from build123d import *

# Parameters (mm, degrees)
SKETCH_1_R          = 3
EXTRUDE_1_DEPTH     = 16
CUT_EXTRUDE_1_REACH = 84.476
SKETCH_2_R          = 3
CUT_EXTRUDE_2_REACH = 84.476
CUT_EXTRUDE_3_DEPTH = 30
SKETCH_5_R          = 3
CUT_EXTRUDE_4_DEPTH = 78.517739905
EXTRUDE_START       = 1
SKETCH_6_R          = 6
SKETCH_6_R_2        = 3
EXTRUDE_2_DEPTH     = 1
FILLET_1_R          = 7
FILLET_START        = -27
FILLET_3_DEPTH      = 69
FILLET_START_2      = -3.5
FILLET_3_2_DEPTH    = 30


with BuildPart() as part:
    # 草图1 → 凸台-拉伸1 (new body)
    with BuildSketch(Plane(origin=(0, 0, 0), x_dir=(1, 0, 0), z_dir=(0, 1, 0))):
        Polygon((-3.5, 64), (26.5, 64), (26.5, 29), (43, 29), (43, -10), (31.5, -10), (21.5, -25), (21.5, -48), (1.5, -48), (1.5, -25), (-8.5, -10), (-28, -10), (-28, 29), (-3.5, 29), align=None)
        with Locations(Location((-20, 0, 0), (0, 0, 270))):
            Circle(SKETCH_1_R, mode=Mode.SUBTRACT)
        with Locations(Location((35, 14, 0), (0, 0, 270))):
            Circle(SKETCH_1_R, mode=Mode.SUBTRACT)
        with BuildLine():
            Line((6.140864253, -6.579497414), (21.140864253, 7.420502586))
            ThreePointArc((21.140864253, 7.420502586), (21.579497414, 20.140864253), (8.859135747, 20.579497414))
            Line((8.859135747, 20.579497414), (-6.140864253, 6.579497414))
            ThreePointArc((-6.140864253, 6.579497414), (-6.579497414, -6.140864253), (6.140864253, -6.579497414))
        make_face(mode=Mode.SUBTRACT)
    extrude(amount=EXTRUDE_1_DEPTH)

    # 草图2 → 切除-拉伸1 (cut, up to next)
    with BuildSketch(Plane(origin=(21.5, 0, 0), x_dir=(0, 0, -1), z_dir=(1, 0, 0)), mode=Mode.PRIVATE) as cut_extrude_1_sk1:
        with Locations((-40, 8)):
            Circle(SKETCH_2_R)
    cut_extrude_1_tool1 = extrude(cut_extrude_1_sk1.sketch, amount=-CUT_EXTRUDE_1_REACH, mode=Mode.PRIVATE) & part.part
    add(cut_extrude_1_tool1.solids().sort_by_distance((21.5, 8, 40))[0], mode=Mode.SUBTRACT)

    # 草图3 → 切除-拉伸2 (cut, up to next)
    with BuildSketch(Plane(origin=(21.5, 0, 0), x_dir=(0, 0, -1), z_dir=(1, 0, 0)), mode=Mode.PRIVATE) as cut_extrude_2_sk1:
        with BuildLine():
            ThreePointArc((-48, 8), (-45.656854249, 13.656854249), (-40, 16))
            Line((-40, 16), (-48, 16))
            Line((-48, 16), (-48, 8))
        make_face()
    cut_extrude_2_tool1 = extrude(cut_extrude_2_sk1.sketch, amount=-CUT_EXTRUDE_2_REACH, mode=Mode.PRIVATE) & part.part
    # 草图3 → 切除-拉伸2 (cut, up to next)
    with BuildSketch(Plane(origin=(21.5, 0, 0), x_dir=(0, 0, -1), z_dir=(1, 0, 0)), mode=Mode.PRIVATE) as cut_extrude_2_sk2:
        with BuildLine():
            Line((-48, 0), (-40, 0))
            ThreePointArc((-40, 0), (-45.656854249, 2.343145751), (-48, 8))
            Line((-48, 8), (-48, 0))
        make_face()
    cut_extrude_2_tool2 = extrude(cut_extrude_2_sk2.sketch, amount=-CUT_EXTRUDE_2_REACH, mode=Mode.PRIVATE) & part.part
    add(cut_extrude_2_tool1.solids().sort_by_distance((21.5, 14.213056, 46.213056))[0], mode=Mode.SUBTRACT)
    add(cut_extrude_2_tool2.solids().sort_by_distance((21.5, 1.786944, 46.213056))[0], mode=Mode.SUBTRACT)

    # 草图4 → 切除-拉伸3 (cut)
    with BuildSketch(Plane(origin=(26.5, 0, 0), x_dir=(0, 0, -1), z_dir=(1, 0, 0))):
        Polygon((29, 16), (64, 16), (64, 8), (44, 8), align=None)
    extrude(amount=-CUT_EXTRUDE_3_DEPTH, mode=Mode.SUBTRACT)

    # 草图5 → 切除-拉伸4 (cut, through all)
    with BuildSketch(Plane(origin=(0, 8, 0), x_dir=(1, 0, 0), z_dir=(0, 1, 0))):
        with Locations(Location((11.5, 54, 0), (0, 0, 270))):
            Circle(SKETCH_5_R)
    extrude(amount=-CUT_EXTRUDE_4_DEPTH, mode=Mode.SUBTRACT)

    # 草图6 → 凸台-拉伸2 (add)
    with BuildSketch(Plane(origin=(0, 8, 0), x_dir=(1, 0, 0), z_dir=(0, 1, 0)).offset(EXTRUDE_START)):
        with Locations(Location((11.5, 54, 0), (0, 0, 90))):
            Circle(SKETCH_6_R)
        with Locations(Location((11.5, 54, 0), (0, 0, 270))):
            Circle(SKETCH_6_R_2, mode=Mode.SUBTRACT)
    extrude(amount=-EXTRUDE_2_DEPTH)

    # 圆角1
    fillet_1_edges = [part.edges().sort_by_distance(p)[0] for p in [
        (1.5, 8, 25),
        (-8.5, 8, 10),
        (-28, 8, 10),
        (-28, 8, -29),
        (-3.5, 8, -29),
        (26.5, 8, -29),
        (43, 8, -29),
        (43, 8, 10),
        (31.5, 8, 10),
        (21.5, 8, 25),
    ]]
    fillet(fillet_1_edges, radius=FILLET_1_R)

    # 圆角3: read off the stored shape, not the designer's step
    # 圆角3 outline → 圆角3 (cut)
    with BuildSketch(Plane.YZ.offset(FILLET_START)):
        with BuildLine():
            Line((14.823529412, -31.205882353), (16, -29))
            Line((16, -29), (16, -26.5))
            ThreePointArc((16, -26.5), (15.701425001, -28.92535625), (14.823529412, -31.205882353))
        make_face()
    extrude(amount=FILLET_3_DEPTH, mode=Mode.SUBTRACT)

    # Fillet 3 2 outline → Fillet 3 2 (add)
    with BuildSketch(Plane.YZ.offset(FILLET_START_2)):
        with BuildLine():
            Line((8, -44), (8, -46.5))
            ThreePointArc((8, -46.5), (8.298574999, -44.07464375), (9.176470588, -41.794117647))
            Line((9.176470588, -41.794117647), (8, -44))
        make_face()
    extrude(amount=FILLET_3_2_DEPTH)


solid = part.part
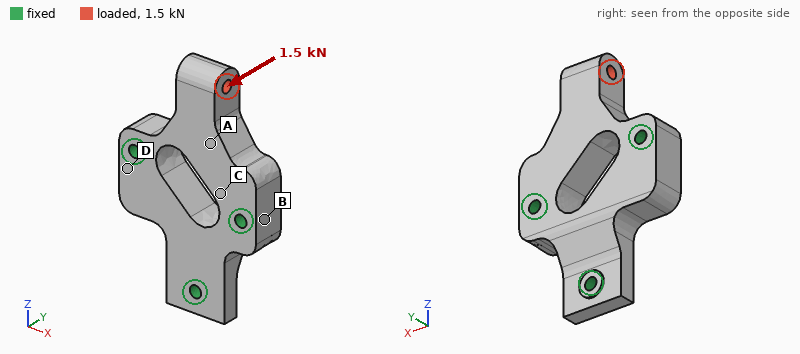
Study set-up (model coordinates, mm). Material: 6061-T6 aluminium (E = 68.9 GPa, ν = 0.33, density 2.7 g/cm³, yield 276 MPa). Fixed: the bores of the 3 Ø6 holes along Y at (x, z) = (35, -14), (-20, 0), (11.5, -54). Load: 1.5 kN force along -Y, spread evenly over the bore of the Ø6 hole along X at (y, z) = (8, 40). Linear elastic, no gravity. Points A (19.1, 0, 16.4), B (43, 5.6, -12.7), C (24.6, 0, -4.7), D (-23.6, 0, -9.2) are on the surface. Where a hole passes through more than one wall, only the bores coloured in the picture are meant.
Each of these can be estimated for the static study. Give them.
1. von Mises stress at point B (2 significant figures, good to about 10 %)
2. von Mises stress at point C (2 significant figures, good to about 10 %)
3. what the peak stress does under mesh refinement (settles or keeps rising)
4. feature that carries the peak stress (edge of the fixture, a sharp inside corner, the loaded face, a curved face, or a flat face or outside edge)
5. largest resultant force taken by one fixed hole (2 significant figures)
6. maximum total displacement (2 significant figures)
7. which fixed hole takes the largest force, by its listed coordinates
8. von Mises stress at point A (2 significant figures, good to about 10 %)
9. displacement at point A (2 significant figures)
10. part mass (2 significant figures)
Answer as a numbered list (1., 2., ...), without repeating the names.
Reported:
1. 14 MPa
2. 47 MPa
3. keeps rising
4. edge of the fixture
5. 1.0 kN
6. 0.17 mm
7. (-20, 0)
8. 39 MPa
9. 0.054 mm
10. 150 g
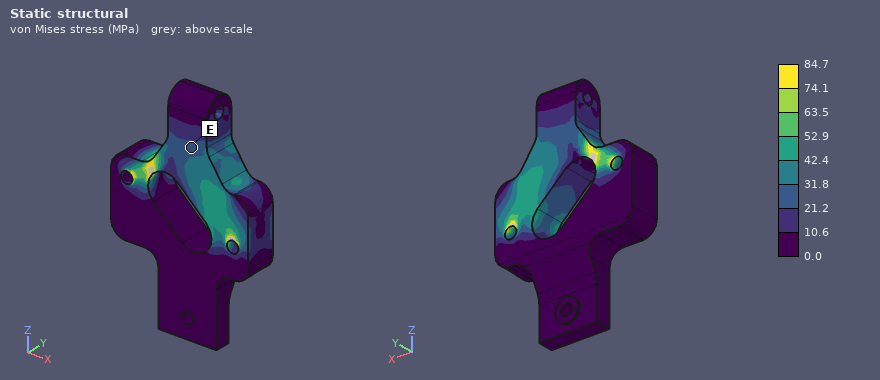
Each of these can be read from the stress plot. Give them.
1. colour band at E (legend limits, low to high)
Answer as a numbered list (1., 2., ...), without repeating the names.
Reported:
1. 21.2 to 31.8 MPa
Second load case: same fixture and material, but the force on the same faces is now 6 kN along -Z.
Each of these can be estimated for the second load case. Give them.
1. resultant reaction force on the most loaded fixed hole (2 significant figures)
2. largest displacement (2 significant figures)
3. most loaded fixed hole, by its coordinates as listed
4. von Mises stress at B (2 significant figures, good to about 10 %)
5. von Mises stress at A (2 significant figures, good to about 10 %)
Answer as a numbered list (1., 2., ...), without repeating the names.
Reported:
1. 4.2 kN
2. 22 µm
3. (35, -14)
4. 4.1 MPa
5. 16 MPa
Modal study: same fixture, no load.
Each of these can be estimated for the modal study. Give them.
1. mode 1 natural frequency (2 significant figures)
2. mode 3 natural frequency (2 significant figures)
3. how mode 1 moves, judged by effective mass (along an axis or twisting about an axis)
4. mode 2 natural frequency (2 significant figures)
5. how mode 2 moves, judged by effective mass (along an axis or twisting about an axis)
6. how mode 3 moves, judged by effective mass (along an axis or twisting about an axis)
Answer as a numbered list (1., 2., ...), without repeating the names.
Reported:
1. 4100 Hz
2. 14 kHz
3. along Y
4. 11 kHz
5. along X
6. along Y
